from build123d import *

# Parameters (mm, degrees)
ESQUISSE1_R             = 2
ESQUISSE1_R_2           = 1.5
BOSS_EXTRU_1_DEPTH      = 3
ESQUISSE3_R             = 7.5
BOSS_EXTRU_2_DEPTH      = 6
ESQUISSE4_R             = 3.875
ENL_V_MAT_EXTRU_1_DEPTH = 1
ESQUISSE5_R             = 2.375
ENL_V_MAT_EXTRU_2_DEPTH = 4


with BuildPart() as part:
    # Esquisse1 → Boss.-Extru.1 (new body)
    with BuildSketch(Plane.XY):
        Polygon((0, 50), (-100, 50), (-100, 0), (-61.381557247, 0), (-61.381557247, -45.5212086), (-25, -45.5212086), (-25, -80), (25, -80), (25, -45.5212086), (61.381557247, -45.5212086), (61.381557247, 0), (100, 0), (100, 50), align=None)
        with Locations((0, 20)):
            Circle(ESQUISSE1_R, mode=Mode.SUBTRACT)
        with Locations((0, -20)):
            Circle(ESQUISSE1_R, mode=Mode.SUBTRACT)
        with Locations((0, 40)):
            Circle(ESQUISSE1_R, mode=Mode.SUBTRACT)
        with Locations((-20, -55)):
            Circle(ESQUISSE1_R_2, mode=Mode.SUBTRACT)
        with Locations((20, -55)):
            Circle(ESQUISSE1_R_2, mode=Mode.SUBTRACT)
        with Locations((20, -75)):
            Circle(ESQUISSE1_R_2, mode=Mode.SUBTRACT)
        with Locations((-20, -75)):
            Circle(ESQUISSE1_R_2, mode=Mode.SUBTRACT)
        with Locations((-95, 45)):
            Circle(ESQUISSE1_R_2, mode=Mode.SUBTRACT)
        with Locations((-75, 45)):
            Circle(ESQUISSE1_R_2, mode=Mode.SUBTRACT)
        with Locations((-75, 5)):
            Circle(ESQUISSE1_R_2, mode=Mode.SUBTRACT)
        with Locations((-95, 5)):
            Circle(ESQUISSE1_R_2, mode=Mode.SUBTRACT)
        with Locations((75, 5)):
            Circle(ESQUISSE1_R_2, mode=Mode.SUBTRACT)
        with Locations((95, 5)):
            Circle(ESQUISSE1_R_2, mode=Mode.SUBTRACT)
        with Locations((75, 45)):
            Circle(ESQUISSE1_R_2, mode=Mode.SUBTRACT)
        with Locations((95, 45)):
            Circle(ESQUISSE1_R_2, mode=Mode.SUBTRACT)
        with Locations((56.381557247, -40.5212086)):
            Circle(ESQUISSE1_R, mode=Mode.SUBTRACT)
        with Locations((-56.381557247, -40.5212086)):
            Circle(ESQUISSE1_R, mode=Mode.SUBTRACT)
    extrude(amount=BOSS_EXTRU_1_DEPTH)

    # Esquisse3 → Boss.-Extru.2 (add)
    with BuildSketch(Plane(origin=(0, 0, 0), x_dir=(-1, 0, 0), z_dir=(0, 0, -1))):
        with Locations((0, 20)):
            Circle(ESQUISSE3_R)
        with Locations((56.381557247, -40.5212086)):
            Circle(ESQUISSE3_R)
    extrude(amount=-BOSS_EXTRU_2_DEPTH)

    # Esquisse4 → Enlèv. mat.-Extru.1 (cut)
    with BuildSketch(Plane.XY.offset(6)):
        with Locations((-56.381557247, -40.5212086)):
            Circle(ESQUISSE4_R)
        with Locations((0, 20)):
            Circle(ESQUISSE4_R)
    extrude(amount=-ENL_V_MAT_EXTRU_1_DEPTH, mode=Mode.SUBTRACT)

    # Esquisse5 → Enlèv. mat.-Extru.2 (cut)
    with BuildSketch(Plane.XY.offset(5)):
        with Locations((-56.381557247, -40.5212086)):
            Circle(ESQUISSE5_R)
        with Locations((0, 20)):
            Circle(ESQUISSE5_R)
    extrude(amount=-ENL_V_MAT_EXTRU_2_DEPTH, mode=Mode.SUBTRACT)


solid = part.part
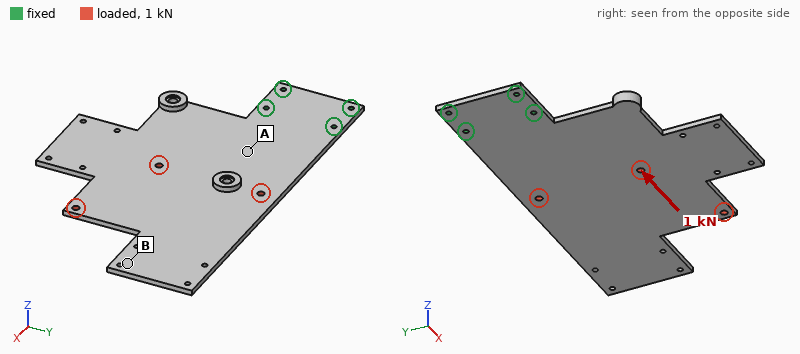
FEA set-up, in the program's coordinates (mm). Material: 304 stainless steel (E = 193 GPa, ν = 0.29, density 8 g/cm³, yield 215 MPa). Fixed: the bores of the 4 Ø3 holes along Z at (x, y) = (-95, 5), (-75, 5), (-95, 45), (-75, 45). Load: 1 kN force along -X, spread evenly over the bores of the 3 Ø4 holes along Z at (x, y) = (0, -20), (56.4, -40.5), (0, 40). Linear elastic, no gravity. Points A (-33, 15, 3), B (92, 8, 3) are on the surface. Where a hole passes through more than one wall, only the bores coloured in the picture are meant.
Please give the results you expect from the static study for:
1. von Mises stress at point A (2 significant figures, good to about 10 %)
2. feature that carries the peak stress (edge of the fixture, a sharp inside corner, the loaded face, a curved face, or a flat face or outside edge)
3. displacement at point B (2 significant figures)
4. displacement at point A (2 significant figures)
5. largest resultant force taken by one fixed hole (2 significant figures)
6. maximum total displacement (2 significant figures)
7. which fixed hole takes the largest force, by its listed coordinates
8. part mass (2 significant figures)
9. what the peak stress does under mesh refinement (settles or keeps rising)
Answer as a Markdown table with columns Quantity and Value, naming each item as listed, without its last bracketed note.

| Quantity | Value |
|---|---|
| von Mises stress at point A | 8.7 MPa |
| feature that carries the peak stress | edge of the fixture |
| displacement at point B | 32 µm |
| displacement at point A | 6.1 µm |
| largest resultant force taken by one fixed hole | 1.1 kN |
| maximum total displacement | 34 µm |
| which fixed hole takes the largest force, by its listed coordinates | (-75, 5) |
| part mass | 420 g |
| what the peak stress does under mesh refinement | keeps rising |
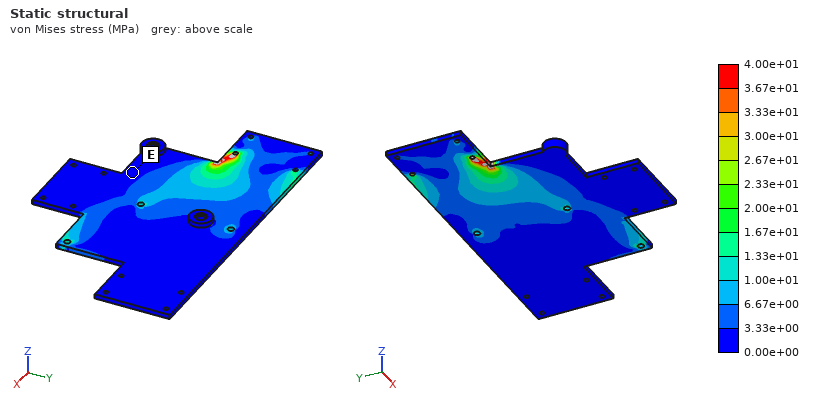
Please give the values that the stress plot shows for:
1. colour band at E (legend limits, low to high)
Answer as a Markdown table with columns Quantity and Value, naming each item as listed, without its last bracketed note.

| Quantity | Value |
|---|---|
| colour band at E | 0.00e+00 to 3.33e+00 MPa |
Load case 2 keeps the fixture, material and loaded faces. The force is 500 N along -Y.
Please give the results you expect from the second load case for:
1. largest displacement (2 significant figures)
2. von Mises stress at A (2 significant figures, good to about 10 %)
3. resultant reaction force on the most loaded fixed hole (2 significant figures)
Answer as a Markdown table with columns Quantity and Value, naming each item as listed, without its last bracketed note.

| Quantity | Value |
|---|---|
| largest displacement | 47 µm |
| von Mises stress at A | 9.6 MPa |
| resultant reaction force on the most loaded fixed hole | 1.1 kN |
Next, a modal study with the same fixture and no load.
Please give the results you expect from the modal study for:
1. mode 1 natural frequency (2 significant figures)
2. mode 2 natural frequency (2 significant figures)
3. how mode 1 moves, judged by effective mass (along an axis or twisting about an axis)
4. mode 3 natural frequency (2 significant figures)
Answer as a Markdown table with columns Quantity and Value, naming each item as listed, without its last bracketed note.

| Quantity | Value |
|---|---|
| mode 1 natural frequency | 71 Hz |
| mode 2 natural frequency | 190 Hz |
| how mode 1 moves, judged by effective mass | along Z |
| mode 3 natural frequency | 540 Hz |
